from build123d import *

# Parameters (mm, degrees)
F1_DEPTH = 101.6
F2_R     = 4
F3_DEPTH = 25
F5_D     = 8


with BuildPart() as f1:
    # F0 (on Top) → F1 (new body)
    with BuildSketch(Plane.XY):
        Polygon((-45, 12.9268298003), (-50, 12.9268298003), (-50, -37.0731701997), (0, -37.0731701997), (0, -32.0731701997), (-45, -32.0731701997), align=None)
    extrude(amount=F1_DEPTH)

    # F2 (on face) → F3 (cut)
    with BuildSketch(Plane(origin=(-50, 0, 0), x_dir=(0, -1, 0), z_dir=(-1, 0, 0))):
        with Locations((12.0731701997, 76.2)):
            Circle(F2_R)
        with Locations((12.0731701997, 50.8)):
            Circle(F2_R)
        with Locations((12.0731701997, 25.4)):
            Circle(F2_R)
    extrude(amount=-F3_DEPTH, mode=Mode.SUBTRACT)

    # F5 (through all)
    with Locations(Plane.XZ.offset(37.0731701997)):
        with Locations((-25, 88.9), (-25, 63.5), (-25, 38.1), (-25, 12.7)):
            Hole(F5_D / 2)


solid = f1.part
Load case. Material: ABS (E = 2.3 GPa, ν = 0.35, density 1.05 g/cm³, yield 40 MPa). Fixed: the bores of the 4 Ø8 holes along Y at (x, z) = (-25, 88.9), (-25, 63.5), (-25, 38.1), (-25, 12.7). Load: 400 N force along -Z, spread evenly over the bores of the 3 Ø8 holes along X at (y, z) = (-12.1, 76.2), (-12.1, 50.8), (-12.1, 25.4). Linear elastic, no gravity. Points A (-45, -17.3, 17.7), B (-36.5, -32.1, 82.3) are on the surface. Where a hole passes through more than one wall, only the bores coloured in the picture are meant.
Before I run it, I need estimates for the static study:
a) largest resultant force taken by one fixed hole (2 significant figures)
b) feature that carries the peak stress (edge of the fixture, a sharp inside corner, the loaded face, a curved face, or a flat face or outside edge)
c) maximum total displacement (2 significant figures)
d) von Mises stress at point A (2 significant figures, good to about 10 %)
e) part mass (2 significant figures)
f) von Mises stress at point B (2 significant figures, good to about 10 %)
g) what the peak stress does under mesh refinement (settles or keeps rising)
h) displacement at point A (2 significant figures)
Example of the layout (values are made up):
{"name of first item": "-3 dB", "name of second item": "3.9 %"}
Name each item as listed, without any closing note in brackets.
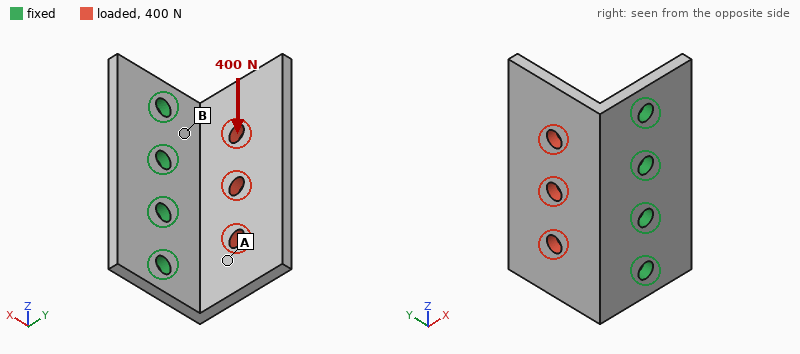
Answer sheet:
{"largest resultant force taken by one fixed hole": "170 N", "feature that carries the peak stress": "edge of the fixture", "maximum total displacement": "0.74 mm", "von Mises stress at point A": "2.9 MPa", "part mass": "49 g", "von Mises stress at point B": "6.0 MPa", "what the peak stress does under mesh refinement": "keeps rising", "displacement at point A": "0.33 mm"}
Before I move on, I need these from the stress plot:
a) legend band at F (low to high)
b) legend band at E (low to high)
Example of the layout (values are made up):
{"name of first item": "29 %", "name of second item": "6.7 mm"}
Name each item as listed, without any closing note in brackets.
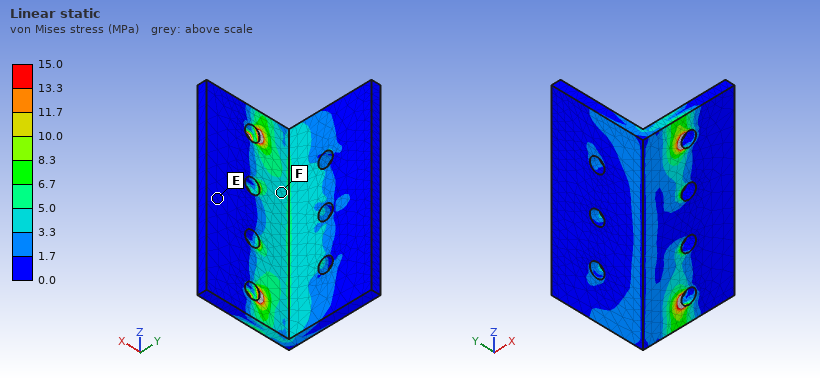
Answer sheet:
{"legend band at F": "3.3 to 5.0 MPa", "legend band at E": "0.0 to 1.7 MPa"}
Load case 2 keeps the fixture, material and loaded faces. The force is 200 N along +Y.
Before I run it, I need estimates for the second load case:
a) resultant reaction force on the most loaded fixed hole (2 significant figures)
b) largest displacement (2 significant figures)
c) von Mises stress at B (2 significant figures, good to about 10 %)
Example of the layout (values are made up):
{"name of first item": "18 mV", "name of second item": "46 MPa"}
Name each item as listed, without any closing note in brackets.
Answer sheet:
{"resultant reaction force on the most loaded fixed hole": "53 N", "largest displacement": "0.82 mm", "von Mises stress at B": "4.5 MPa"}
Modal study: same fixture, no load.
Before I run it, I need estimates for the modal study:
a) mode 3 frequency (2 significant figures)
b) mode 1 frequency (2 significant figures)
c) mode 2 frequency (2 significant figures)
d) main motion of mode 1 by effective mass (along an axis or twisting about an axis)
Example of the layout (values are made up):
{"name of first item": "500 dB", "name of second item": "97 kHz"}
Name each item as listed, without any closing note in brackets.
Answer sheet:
{"mode 3 frequency": "1000 Hz", "mode 1 frequency": "330 Hz", "mode 2 frequency": "560 Hz", "main motion of mode 1 by effective mass": "along X"}
